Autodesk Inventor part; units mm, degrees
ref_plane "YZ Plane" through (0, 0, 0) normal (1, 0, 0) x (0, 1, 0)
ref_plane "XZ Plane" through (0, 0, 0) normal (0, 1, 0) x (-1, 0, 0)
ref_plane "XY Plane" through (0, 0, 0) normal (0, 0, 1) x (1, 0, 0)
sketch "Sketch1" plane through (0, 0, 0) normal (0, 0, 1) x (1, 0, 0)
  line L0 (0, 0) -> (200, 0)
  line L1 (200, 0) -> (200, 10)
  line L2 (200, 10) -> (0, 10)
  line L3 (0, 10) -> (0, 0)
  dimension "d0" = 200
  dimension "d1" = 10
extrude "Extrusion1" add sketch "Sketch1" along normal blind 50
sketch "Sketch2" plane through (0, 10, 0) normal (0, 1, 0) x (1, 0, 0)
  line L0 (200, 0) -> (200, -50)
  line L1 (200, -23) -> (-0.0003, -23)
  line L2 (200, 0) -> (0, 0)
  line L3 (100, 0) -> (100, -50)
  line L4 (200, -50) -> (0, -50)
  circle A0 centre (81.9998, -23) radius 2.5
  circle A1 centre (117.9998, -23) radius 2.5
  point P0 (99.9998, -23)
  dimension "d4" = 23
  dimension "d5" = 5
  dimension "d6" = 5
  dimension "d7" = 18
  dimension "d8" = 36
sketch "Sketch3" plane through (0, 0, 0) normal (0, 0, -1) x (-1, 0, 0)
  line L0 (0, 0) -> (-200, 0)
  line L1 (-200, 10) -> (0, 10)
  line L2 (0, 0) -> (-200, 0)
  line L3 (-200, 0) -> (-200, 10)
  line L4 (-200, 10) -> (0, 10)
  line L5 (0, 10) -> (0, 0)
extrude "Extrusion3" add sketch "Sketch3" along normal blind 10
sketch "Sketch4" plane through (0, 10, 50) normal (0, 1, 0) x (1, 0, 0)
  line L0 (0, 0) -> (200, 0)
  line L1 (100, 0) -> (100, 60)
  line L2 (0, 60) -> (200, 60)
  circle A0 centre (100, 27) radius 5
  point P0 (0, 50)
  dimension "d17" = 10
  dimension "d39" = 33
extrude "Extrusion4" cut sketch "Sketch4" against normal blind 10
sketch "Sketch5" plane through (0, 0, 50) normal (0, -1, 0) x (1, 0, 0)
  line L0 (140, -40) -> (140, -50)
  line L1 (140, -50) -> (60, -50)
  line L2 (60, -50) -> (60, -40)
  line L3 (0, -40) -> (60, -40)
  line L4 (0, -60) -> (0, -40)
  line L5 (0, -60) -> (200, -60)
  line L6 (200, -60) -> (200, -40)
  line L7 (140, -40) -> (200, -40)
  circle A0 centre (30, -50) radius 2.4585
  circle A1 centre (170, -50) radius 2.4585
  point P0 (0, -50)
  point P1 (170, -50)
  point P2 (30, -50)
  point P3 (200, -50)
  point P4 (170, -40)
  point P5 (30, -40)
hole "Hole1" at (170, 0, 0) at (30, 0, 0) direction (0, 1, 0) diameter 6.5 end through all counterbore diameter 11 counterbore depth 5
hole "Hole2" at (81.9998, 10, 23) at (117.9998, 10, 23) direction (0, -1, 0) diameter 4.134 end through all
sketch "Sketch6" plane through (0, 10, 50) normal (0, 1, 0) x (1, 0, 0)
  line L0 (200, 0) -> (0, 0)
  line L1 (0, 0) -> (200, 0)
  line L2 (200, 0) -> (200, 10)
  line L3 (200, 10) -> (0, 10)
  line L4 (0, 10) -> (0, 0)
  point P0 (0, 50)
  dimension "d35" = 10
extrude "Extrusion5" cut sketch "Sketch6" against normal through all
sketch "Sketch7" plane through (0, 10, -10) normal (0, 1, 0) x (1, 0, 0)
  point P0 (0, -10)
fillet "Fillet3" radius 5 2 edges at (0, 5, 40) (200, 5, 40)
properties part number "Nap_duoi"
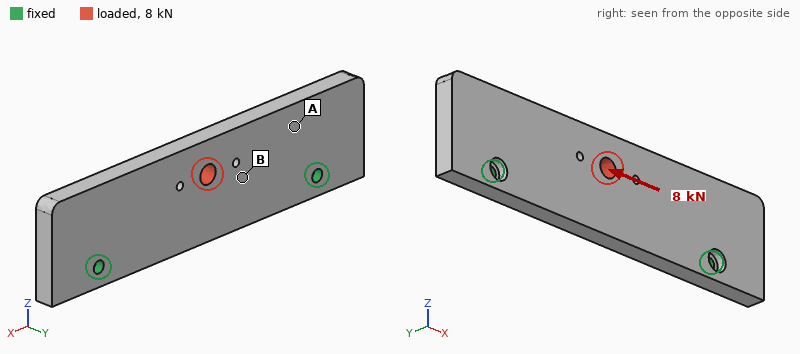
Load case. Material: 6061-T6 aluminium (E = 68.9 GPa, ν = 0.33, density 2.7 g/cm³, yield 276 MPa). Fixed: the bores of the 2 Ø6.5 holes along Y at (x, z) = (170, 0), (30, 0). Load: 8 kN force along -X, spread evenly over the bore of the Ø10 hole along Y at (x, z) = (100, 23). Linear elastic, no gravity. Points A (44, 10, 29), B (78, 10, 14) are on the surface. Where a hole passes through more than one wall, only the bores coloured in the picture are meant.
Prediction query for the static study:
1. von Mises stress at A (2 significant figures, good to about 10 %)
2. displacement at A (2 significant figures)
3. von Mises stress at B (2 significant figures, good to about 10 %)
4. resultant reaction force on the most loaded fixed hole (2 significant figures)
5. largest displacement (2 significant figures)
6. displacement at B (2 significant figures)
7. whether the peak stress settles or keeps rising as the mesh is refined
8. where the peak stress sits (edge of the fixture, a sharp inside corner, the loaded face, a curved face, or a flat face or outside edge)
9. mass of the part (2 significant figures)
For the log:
8.1 MPa
14 µm
17 MPa
4.2 kN
22 µm
15 µm
keeps rising
edge of the fixture
260 g
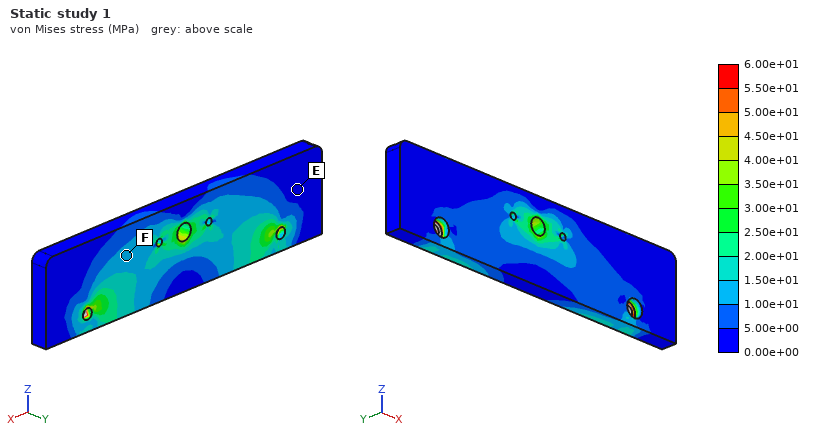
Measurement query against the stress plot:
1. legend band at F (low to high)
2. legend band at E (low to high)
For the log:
1.00e+01 to 1.50e+01 MPa
0.00e+00 to 5.00e+00 MPa
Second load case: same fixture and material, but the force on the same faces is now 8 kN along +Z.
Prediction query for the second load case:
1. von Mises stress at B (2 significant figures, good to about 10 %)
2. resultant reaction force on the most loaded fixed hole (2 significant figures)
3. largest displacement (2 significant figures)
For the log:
23 MPa
5.3 kN
0.10 mm
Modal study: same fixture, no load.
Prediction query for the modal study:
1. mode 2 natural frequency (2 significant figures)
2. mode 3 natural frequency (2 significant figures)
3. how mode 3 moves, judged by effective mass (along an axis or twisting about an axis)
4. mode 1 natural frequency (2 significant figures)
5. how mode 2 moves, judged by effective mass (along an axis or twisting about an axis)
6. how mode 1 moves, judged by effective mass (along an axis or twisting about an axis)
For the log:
2400 Hz
2900 Hz
twisting about Z
1500 Hz
twisting about X
along Y
